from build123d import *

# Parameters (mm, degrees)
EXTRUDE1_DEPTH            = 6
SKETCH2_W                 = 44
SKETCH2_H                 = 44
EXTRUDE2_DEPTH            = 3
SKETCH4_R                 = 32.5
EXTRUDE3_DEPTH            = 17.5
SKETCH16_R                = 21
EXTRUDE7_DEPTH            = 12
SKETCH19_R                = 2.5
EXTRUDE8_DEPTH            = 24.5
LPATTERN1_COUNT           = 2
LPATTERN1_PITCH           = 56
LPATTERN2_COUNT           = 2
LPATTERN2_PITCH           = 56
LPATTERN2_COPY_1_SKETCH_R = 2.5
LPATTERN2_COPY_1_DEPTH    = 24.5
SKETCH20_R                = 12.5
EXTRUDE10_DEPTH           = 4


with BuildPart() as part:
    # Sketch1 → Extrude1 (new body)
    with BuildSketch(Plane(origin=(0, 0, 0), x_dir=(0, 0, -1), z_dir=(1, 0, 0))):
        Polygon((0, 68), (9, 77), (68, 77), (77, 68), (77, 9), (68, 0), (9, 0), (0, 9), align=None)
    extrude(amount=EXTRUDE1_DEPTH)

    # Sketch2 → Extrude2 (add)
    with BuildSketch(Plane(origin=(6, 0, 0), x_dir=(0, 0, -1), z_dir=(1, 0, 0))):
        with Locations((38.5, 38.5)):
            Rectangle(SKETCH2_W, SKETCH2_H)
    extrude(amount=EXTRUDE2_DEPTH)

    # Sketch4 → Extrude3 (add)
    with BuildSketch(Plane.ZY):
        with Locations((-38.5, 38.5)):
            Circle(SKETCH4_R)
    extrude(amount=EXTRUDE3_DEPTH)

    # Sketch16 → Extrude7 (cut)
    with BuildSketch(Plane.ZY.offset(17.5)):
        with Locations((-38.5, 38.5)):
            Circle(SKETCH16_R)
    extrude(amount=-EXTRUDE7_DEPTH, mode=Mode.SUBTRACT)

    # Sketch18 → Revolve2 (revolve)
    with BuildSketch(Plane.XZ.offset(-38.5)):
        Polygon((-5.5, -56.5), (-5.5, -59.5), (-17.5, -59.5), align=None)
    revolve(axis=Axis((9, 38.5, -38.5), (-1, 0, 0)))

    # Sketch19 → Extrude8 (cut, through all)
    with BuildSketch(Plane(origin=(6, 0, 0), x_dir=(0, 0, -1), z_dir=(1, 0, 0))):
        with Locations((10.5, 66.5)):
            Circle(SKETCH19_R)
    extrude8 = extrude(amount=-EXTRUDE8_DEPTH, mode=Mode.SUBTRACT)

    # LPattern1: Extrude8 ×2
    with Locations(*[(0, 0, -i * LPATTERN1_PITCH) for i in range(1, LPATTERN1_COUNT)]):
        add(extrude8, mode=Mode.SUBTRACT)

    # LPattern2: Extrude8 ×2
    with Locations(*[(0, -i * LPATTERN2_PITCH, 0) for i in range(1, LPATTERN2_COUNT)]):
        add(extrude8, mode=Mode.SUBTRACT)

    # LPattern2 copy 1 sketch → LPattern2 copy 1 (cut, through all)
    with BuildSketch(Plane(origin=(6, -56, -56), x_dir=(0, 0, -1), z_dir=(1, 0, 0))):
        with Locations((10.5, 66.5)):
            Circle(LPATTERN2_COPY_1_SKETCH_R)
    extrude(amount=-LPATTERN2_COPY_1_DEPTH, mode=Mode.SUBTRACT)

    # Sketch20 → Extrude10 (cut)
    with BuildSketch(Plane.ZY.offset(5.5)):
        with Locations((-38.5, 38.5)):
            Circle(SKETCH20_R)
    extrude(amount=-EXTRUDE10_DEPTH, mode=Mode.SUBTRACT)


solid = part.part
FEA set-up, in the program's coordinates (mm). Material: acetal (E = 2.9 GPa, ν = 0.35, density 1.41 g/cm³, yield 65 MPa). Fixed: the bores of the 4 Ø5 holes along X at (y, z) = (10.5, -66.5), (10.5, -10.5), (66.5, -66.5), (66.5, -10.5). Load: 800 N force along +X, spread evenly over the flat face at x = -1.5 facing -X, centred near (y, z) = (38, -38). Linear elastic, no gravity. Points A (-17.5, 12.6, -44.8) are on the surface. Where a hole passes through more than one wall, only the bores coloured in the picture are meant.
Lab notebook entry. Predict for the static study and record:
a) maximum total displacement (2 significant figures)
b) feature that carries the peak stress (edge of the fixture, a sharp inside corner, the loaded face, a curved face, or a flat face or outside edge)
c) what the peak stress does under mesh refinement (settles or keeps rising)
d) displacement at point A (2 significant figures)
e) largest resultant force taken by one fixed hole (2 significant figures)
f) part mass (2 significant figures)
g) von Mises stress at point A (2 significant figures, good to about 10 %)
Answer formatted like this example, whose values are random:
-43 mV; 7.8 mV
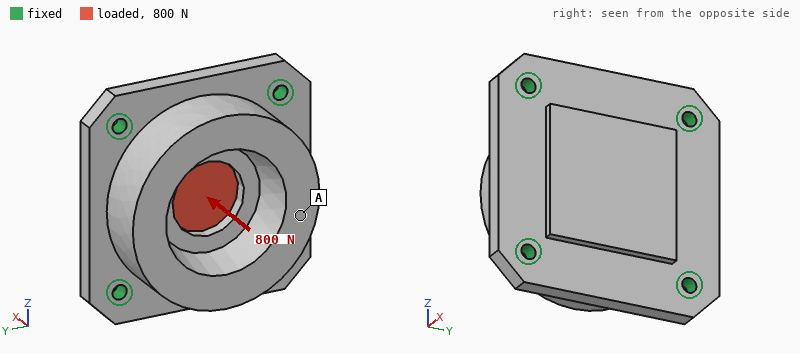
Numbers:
74 µm; edge of the fixture; keeps rising; 40 µm; 220 N; 120 g; 1.4 MPa
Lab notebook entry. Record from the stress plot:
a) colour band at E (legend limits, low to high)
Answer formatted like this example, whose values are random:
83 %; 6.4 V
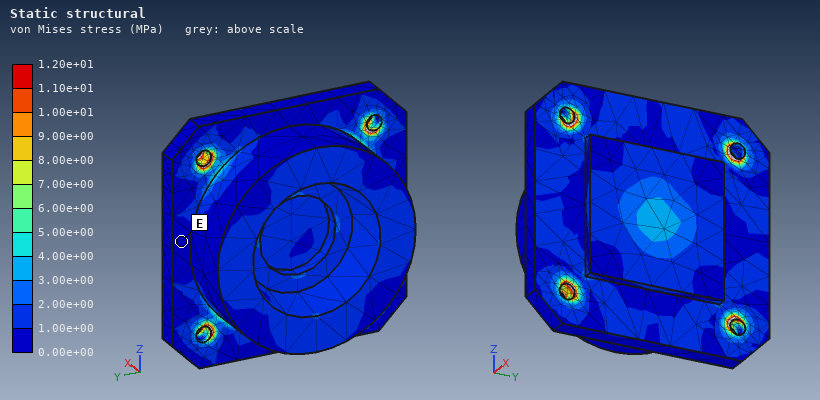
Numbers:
0.00e+00 to 1.00e+00 MPa
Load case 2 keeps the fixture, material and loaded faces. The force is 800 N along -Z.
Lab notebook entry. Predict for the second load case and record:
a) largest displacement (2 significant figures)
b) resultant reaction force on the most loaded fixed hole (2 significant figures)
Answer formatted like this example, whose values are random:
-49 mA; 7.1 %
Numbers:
27 µm; 220 N
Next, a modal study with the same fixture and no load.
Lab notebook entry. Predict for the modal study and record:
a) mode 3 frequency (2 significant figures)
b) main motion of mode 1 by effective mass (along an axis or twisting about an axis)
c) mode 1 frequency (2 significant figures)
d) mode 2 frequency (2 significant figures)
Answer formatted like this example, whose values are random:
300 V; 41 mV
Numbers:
2900 Hz; along X; 2300 Hz; 2900 Hz
